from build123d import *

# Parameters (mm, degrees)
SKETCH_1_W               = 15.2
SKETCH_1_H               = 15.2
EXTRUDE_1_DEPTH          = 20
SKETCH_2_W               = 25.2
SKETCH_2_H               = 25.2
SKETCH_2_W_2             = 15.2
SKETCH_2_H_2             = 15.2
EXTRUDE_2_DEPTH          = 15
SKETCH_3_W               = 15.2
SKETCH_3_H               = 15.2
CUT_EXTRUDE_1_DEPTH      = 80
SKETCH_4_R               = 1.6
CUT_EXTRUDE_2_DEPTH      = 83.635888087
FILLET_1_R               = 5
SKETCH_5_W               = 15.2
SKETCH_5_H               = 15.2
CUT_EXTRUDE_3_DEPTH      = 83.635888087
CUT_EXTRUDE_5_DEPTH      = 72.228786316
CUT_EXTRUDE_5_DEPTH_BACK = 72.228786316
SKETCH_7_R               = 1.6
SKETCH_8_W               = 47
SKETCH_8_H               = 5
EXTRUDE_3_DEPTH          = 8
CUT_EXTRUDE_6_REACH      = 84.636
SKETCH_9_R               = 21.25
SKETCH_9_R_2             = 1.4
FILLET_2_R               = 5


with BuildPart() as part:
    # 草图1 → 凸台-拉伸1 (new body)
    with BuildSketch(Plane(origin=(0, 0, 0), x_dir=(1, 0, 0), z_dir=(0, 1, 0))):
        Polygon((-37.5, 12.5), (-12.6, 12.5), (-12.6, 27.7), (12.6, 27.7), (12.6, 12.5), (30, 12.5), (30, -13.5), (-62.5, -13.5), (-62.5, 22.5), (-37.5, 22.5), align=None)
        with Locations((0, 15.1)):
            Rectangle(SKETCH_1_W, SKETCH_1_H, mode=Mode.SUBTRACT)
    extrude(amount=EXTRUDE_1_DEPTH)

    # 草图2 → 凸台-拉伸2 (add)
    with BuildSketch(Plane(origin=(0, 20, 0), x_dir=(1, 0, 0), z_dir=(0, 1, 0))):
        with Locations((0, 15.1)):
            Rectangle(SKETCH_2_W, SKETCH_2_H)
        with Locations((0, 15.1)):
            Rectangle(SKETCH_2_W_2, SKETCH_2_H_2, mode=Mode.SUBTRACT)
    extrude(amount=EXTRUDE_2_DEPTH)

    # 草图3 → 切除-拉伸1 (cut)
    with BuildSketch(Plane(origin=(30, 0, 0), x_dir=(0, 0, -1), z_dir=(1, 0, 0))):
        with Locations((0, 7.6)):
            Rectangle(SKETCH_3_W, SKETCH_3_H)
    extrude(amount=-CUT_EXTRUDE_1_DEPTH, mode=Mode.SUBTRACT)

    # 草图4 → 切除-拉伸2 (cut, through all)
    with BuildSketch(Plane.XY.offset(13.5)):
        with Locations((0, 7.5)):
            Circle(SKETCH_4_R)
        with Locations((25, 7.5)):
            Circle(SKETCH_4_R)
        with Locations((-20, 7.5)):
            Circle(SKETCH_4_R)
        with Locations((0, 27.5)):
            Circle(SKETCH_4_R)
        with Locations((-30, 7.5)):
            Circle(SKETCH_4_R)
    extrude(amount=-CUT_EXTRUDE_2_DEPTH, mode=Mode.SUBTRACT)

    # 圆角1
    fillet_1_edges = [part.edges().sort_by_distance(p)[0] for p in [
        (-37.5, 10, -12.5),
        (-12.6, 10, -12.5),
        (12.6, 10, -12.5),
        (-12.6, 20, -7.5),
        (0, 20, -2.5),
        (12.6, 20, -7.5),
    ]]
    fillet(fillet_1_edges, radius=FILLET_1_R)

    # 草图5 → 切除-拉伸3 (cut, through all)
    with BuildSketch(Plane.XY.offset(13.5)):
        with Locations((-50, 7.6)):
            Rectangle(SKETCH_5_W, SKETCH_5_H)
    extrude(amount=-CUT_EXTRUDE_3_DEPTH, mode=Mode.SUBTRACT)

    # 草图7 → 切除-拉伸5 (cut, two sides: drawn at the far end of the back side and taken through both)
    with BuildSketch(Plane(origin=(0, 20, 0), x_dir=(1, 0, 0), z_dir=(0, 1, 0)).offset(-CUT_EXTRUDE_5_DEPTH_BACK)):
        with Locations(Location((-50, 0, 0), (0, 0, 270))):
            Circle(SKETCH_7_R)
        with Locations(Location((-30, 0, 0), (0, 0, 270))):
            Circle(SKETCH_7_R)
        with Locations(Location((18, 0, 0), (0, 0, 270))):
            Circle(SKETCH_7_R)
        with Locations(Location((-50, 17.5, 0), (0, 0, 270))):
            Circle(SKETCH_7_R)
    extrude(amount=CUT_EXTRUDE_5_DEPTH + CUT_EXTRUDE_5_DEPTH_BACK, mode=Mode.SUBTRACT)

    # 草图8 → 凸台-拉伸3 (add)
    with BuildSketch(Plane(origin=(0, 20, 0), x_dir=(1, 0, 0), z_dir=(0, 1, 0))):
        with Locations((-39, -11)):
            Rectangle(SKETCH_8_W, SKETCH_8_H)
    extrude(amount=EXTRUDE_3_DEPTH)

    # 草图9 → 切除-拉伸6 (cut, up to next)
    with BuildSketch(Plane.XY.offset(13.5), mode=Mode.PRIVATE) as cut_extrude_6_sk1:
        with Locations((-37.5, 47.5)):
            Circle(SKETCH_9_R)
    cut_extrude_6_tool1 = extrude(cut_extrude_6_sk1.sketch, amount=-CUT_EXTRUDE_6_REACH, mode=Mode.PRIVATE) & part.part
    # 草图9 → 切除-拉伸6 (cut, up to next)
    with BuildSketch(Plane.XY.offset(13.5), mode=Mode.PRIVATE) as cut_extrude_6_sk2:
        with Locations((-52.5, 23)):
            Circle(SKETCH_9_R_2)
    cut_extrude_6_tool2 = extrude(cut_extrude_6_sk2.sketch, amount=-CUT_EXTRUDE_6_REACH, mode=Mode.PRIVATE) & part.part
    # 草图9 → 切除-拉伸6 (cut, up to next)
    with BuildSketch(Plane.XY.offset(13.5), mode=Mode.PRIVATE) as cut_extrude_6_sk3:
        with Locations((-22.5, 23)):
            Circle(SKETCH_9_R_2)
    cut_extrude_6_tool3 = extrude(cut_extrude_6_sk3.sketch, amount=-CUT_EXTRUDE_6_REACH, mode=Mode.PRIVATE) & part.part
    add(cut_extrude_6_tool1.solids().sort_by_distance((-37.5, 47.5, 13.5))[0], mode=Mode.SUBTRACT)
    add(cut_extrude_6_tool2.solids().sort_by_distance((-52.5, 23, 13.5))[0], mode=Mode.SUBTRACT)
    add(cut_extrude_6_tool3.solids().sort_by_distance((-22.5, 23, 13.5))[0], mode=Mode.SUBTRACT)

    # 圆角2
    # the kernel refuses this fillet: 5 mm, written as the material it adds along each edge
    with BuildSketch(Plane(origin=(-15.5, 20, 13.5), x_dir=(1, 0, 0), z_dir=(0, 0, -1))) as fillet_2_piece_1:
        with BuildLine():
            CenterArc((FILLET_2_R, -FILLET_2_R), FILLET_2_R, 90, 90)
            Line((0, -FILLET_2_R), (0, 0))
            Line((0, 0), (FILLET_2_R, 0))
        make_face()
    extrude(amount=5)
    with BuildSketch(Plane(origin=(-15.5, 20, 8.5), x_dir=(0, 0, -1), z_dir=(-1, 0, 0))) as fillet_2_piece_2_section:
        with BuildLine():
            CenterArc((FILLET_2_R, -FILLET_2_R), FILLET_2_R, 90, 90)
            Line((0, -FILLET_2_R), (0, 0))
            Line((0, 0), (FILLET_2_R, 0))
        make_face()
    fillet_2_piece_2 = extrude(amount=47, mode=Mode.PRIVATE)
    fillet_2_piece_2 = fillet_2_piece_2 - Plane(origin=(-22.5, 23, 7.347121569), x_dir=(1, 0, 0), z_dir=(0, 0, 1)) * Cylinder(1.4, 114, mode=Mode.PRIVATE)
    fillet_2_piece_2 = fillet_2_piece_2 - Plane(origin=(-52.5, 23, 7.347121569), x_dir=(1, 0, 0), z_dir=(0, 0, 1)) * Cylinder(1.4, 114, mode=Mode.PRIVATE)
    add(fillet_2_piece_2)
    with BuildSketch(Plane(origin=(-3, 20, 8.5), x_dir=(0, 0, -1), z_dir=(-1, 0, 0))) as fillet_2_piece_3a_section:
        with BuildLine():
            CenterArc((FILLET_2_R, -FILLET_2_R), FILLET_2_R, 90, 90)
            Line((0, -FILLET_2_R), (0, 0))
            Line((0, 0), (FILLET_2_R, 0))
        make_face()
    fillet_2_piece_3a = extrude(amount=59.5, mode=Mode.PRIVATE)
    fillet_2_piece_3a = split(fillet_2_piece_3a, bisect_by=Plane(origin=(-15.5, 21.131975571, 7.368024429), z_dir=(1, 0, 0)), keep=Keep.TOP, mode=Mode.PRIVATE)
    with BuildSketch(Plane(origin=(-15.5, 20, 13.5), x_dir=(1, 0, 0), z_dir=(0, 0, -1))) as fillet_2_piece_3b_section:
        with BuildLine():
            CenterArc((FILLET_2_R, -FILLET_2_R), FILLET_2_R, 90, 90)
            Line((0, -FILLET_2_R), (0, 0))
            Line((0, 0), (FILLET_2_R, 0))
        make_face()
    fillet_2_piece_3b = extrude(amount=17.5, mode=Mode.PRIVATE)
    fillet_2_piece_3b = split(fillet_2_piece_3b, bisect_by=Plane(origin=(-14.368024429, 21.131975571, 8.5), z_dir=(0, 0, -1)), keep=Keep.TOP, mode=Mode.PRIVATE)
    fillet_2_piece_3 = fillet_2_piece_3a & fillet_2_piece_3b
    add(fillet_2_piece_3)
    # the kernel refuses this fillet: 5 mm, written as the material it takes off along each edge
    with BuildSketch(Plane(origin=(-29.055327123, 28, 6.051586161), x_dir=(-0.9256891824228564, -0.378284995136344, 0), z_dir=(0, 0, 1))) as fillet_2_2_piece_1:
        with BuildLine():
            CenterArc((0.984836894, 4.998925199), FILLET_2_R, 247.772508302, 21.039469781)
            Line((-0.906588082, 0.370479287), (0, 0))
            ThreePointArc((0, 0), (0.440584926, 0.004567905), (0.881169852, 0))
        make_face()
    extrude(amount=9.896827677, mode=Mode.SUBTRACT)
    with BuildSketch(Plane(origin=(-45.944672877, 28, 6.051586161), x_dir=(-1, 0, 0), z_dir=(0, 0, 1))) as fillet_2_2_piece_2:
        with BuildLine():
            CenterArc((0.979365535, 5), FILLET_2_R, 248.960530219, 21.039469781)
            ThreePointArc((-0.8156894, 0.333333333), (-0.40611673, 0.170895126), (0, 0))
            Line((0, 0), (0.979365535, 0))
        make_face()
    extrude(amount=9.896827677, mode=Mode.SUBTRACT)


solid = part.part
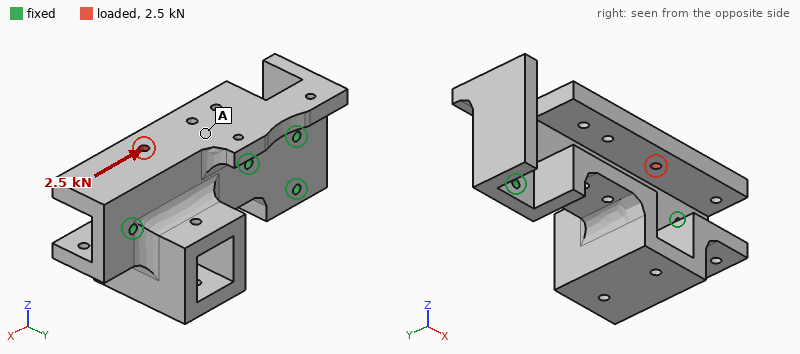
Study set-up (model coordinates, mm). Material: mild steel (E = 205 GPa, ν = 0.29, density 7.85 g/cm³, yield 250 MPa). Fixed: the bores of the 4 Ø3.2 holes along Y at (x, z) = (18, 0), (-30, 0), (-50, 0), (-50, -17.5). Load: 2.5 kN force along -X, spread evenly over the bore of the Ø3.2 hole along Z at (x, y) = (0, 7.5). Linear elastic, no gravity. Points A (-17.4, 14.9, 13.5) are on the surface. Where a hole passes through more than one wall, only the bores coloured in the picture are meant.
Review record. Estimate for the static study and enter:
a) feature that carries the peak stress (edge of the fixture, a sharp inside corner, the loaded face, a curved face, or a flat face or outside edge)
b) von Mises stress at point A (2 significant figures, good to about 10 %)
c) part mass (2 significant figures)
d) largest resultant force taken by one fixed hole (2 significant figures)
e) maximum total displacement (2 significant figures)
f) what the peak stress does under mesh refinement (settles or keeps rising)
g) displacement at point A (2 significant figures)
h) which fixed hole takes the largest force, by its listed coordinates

edge of the fixture
6.6 MPa
310 g
1.3 kN
9.9 µm
keeps rising
1.6 µm
(18, 0)
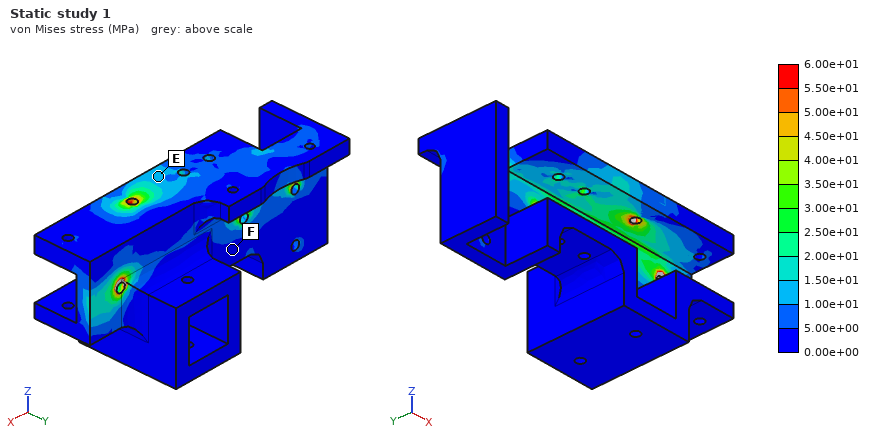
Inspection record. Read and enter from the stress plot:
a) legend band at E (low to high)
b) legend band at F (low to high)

1.00e+01 to 1.50e+01 MPa
0.00e+00 to 5.00e+00 MPa
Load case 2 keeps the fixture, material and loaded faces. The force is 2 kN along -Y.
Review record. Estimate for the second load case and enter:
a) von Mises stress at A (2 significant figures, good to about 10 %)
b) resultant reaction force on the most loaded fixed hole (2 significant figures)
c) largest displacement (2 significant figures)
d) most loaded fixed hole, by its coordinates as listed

23 MPa
1.3 kN
31 µm
(18, 0)
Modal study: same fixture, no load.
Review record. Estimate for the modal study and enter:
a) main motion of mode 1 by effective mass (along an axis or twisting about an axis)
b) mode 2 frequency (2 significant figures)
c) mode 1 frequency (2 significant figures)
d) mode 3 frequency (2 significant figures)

along Y
6000 Hz
2800 Hz
7400 Hz
